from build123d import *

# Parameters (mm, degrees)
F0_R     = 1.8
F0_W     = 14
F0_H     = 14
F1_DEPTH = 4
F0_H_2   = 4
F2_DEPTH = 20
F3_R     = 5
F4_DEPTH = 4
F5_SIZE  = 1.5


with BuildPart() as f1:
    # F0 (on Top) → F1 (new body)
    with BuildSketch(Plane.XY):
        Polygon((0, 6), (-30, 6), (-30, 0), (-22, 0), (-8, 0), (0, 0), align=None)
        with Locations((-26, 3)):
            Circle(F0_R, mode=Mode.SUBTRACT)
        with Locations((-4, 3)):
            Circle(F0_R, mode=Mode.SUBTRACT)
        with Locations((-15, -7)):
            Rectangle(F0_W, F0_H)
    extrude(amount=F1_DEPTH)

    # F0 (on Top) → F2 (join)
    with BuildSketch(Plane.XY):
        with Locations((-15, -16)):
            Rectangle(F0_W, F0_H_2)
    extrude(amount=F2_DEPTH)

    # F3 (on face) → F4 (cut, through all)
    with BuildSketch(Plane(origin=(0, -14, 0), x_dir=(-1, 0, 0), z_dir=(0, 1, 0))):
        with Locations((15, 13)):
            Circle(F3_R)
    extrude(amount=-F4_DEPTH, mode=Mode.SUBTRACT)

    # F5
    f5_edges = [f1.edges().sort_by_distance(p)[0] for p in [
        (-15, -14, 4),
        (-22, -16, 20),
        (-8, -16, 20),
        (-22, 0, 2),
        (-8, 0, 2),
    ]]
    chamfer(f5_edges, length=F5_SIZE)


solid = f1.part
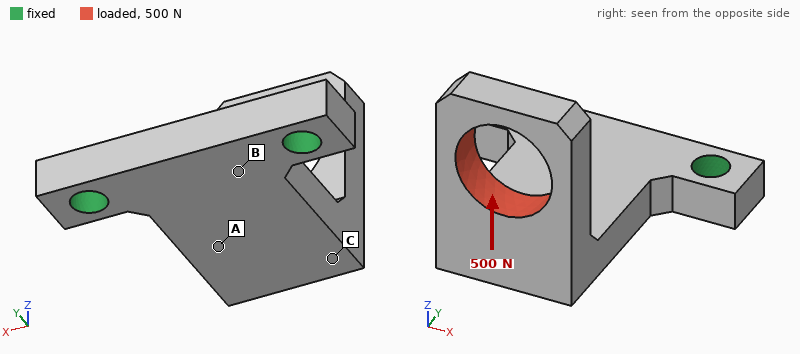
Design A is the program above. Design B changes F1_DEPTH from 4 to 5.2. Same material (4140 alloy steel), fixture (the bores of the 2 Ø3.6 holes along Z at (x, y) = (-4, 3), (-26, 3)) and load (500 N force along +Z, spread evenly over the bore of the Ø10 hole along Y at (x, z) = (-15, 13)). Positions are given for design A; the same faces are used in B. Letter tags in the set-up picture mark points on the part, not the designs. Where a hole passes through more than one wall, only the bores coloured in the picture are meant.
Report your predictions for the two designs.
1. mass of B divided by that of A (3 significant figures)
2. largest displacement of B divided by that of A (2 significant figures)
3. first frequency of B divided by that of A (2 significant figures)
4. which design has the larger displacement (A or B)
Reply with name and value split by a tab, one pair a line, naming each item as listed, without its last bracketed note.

mass of B divided by that of A	1.19
largest displacement of B divided by that of A	0.50
first frequency of B divided by that of A	1.4
which design has the larger displacement	A
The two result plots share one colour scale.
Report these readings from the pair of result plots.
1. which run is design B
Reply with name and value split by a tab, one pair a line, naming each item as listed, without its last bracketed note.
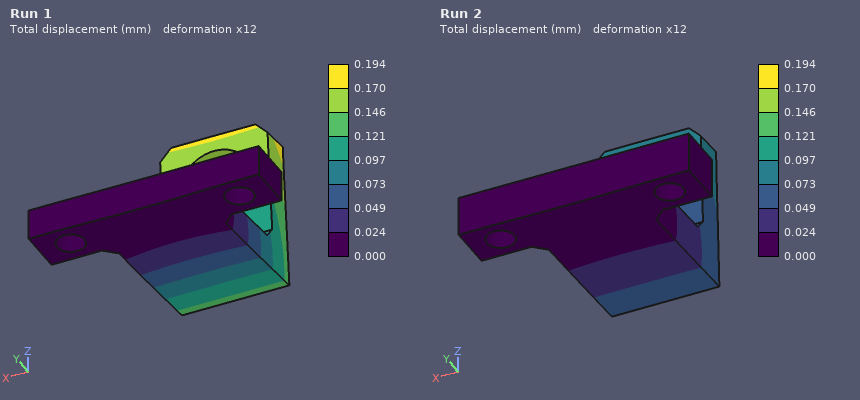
which run is design B	Run 2
